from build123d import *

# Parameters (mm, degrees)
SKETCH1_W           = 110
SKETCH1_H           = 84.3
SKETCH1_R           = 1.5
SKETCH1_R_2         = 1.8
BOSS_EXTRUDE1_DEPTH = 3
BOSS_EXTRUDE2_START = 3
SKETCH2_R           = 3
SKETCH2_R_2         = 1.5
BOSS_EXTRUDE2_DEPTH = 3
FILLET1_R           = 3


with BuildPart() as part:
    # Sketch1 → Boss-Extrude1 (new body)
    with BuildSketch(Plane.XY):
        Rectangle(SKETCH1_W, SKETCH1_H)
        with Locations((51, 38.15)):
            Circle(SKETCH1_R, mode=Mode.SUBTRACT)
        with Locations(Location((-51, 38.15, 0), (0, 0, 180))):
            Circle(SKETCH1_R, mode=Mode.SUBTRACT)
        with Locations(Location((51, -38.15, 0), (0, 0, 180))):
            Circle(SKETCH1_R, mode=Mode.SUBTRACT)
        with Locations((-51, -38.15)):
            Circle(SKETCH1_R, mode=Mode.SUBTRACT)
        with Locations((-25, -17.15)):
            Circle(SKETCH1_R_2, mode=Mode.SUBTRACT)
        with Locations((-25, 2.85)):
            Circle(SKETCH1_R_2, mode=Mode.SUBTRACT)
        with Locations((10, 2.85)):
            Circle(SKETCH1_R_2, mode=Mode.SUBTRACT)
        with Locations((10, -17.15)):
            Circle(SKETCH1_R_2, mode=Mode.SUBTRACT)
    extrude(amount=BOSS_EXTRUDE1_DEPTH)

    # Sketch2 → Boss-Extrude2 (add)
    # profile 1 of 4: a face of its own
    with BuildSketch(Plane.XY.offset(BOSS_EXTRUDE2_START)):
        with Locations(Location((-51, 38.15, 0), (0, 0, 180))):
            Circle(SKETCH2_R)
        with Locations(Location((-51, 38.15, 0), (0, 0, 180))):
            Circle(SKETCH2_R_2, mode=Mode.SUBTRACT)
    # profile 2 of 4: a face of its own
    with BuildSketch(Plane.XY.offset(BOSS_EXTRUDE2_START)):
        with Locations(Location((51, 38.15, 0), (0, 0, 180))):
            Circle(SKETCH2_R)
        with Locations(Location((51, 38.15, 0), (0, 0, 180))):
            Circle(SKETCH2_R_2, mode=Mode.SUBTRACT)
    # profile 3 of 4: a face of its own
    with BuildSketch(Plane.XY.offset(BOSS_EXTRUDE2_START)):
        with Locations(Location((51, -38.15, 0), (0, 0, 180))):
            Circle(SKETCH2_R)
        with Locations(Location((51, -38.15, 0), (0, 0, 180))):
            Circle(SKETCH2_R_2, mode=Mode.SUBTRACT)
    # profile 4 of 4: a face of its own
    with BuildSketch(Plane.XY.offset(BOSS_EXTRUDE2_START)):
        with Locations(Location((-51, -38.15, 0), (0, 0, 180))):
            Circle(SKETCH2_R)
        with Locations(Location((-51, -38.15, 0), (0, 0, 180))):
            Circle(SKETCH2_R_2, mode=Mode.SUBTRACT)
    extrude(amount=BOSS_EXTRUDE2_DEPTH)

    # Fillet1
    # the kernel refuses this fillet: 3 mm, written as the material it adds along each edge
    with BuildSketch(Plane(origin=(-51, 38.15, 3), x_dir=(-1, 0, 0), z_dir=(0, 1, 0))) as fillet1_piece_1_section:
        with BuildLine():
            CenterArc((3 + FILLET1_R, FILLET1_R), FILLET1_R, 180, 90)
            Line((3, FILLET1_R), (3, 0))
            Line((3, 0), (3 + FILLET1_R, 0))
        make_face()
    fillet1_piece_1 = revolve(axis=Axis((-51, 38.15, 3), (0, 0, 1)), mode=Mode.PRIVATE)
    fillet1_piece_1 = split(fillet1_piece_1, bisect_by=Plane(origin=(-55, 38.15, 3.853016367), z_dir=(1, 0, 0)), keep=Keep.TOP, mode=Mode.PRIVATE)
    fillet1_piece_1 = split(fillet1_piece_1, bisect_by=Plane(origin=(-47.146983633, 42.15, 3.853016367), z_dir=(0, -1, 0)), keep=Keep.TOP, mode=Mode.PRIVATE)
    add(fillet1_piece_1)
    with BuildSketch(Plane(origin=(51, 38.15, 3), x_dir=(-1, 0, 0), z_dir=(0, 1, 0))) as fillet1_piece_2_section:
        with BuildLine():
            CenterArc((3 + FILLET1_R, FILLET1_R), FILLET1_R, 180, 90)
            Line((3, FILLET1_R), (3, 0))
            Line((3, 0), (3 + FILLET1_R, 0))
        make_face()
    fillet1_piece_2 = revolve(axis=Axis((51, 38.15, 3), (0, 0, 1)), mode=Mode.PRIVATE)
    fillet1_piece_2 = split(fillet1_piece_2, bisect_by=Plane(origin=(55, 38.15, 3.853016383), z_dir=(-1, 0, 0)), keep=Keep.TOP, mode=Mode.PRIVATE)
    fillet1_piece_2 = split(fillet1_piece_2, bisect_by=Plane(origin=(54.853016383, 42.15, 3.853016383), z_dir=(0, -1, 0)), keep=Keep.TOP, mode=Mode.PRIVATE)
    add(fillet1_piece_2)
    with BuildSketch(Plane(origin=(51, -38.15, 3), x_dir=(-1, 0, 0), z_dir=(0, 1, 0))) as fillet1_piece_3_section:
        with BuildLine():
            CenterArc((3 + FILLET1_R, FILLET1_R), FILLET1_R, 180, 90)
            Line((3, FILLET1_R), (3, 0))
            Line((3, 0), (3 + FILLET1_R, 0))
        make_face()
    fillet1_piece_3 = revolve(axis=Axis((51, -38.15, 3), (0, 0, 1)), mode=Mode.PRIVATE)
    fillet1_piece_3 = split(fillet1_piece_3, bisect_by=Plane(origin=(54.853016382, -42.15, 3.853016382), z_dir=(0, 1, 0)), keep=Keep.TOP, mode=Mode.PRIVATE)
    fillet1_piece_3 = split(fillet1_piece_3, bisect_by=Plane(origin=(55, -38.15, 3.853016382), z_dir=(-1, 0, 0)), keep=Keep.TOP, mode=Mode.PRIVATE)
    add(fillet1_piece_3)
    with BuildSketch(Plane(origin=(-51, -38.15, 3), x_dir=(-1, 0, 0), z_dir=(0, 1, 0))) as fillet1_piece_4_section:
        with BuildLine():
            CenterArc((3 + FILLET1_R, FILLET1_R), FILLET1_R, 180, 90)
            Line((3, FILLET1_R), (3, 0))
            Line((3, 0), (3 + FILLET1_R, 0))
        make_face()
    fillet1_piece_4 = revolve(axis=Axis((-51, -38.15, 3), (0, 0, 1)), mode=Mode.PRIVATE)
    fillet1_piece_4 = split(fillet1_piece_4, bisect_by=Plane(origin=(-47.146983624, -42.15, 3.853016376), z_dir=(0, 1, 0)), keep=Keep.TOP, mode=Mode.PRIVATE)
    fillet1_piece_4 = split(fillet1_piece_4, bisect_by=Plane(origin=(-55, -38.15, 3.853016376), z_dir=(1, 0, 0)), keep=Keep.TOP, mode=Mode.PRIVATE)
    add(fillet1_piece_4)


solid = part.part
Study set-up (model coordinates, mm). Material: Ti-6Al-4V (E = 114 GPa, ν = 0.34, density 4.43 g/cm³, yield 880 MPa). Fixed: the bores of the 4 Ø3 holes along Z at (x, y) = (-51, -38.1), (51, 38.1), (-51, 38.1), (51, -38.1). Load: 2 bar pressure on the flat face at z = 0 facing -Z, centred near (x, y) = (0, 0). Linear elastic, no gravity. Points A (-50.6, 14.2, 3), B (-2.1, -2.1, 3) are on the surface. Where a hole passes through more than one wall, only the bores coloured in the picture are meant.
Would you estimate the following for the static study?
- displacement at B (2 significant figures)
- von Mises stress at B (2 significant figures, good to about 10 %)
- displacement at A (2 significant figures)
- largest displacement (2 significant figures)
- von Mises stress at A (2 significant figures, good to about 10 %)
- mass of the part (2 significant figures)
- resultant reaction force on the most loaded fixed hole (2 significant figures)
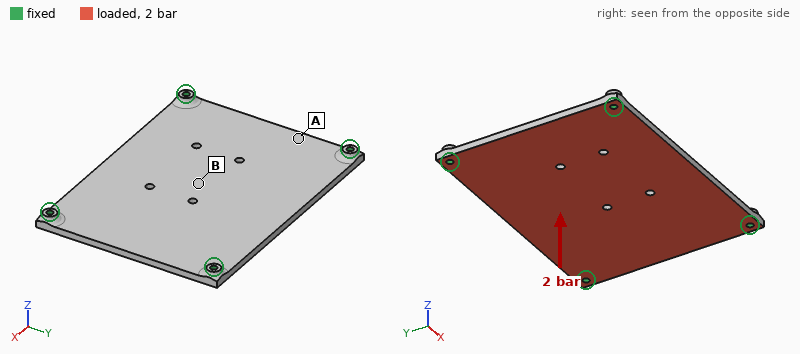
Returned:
0.37 mm
61 MPa
0.070 mm
0.37 mm
28 MPa
120 g
540 N
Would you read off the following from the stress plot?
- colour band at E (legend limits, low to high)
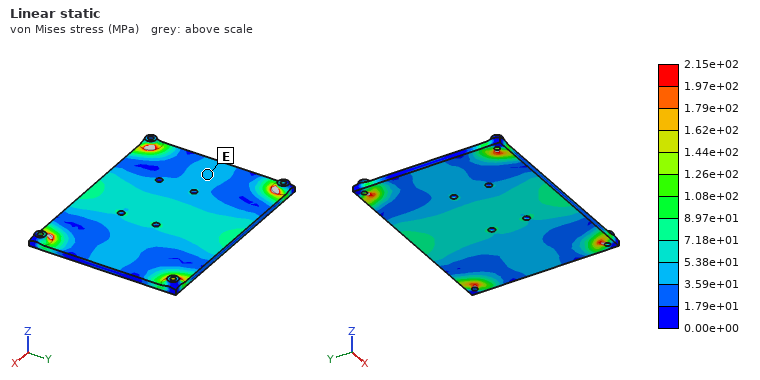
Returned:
3.59e+01 to 5.38e+01 MPa
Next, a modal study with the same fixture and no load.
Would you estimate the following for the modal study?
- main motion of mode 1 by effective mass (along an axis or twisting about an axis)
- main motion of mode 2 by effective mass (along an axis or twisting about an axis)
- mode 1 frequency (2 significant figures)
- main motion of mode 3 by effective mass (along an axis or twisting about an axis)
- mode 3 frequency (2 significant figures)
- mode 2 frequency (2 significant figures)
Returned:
along Z
twisting about X
1200 Hz
twisting about Y
2700 Hz
2000 Hz
